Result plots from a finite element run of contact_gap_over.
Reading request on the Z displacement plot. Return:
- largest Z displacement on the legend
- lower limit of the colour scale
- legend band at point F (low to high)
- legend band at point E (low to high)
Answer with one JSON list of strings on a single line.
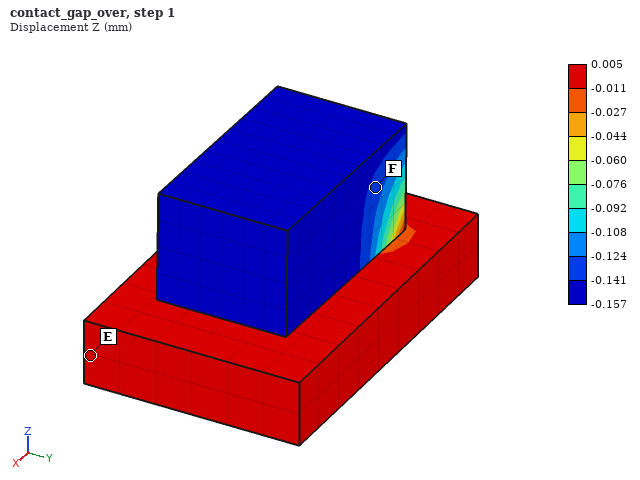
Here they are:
["0.005 mm", "-0.157 mm", "-0.141 to -0.124 mm", "-0.011 to 0.005 mm"]
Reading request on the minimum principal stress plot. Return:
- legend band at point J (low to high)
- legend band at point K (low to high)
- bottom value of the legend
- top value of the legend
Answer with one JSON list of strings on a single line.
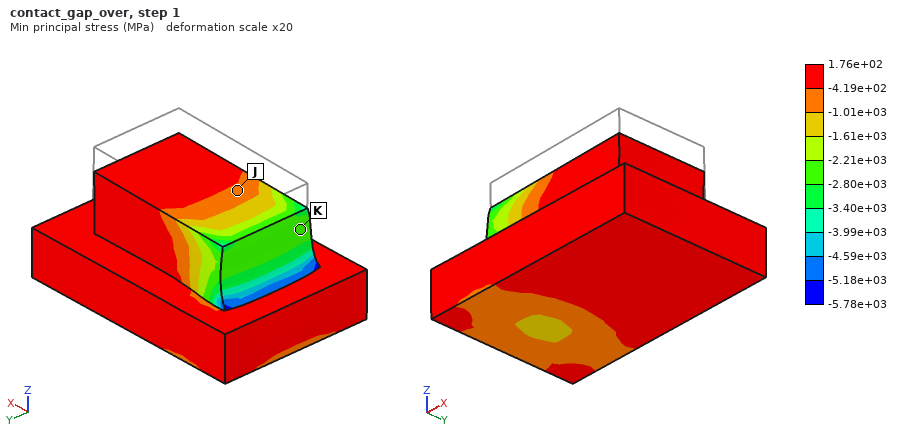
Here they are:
["-1.01e+03 to -4.19e+02 MPa", "-2.80e+03 to -2.21e+03 MPa", "-5.78e+03 MPa", "1.76e+02 MPa"]
